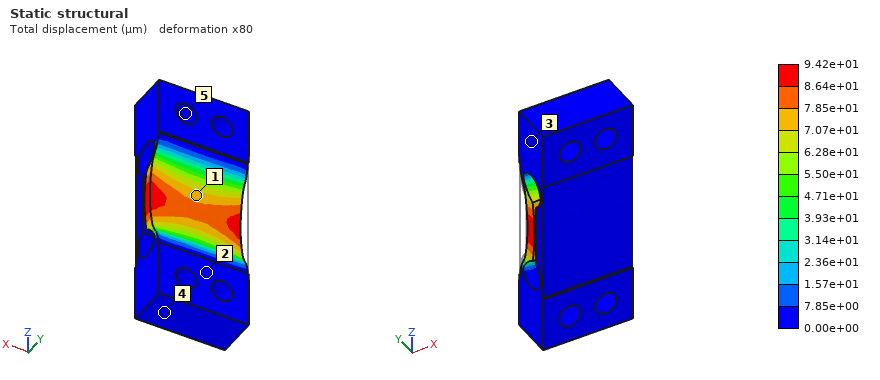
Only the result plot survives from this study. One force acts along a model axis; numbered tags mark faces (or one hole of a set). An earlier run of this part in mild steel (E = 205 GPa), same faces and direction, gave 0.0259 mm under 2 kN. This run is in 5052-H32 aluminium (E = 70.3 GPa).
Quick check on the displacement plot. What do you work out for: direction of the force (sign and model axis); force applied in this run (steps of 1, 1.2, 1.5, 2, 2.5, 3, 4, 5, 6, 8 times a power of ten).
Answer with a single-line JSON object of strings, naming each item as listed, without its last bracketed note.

{"direction of the force": "-Y", "force applied in this run": "2.5 kN"}
